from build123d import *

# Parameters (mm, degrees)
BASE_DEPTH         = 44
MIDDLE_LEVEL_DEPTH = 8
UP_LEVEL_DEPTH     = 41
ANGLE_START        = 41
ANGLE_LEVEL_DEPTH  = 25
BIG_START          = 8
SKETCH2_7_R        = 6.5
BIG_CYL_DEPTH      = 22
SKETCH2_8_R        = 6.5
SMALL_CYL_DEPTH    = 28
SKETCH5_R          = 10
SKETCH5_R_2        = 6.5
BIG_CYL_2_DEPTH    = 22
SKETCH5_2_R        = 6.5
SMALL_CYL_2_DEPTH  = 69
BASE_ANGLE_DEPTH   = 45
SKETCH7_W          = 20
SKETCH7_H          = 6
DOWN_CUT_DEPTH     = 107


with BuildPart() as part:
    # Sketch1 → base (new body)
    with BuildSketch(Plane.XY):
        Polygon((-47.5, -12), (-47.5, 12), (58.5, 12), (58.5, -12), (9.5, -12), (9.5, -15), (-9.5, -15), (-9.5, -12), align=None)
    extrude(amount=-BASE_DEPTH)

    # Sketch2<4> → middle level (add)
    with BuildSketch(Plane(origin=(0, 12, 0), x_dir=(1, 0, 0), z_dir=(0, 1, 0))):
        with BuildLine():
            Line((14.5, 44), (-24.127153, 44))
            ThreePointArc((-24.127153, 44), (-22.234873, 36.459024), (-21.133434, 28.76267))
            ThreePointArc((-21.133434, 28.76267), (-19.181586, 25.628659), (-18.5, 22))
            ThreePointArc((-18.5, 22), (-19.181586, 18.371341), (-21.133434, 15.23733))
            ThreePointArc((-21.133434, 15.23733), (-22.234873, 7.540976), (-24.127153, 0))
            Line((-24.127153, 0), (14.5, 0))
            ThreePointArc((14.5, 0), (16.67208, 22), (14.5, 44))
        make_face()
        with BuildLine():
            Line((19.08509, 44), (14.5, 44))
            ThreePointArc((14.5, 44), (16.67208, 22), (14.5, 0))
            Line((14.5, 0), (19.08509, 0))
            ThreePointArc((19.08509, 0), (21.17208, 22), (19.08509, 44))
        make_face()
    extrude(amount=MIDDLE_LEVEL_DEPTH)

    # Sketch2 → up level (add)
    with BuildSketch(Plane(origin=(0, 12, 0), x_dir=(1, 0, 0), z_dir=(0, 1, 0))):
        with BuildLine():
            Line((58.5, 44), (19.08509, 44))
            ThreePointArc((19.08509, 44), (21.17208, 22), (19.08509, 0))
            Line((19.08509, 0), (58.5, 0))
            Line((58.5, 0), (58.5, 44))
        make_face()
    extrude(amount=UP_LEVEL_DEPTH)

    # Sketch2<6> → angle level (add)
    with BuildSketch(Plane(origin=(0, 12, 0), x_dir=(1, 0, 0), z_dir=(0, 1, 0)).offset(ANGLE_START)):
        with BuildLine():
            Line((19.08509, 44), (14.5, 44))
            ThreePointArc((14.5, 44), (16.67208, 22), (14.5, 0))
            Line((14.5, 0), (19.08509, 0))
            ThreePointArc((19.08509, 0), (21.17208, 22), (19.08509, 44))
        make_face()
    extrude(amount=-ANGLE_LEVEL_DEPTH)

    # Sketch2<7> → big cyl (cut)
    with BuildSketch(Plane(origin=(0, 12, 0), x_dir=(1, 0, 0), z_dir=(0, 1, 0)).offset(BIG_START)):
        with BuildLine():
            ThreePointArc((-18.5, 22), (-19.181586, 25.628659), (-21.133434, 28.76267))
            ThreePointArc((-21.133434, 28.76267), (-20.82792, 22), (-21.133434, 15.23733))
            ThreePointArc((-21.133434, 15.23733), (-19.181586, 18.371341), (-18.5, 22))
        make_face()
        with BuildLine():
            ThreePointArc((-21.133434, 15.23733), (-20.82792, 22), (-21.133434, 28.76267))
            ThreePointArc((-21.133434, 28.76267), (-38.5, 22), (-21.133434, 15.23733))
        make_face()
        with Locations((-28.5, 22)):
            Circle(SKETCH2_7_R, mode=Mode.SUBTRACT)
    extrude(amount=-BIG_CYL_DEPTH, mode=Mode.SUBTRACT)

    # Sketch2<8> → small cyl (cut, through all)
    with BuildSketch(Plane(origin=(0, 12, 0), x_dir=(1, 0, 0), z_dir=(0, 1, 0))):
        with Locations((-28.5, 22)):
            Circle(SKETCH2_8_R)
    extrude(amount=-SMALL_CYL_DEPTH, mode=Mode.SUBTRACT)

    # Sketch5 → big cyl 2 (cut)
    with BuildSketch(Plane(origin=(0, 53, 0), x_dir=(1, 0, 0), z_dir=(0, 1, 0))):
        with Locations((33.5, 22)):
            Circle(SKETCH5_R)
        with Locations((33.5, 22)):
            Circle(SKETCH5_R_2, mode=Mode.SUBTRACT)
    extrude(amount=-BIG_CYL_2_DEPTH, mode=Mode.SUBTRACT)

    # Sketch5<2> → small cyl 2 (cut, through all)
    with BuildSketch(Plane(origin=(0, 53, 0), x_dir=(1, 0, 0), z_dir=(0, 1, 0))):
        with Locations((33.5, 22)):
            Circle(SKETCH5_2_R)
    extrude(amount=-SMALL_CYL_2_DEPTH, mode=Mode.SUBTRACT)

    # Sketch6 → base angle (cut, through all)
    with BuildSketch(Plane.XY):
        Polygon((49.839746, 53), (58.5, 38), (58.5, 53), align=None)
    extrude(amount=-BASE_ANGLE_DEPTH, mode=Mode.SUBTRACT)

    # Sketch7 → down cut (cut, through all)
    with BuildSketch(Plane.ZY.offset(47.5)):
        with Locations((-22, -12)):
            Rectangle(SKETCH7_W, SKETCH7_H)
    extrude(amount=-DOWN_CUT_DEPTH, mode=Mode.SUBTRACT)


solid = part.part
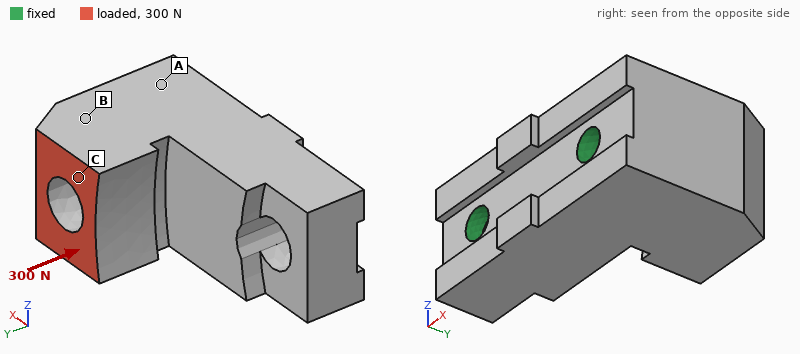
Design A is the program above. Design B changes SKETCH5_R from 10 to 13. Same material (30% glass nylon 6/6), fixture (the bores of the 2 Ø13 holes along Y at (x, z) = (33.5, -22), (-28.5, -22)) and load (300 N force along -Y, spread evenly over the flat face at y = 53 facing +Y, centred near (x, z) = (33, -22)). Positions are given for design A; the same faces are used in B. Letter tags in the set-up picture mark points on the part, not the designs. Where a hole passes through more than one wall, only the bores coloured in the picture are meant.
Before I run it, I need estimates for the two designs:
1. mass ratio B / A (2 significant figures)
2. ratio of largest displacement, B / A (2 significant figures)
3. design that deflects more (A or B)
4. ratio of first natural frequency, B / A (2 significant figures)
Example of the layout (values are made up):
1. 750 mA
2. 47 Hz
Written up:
1. 0.97
2. 1.3
3. B
4. 1.0
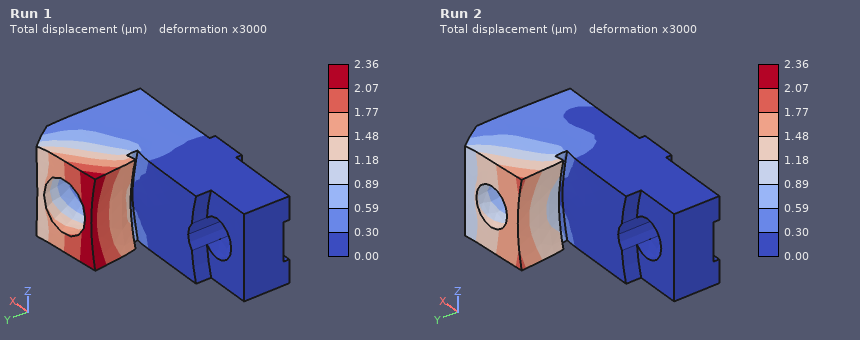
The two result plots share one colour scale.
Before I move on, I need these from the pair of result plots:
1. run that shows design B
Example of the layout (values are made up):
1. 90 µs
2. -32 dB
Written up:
1. Run 1
